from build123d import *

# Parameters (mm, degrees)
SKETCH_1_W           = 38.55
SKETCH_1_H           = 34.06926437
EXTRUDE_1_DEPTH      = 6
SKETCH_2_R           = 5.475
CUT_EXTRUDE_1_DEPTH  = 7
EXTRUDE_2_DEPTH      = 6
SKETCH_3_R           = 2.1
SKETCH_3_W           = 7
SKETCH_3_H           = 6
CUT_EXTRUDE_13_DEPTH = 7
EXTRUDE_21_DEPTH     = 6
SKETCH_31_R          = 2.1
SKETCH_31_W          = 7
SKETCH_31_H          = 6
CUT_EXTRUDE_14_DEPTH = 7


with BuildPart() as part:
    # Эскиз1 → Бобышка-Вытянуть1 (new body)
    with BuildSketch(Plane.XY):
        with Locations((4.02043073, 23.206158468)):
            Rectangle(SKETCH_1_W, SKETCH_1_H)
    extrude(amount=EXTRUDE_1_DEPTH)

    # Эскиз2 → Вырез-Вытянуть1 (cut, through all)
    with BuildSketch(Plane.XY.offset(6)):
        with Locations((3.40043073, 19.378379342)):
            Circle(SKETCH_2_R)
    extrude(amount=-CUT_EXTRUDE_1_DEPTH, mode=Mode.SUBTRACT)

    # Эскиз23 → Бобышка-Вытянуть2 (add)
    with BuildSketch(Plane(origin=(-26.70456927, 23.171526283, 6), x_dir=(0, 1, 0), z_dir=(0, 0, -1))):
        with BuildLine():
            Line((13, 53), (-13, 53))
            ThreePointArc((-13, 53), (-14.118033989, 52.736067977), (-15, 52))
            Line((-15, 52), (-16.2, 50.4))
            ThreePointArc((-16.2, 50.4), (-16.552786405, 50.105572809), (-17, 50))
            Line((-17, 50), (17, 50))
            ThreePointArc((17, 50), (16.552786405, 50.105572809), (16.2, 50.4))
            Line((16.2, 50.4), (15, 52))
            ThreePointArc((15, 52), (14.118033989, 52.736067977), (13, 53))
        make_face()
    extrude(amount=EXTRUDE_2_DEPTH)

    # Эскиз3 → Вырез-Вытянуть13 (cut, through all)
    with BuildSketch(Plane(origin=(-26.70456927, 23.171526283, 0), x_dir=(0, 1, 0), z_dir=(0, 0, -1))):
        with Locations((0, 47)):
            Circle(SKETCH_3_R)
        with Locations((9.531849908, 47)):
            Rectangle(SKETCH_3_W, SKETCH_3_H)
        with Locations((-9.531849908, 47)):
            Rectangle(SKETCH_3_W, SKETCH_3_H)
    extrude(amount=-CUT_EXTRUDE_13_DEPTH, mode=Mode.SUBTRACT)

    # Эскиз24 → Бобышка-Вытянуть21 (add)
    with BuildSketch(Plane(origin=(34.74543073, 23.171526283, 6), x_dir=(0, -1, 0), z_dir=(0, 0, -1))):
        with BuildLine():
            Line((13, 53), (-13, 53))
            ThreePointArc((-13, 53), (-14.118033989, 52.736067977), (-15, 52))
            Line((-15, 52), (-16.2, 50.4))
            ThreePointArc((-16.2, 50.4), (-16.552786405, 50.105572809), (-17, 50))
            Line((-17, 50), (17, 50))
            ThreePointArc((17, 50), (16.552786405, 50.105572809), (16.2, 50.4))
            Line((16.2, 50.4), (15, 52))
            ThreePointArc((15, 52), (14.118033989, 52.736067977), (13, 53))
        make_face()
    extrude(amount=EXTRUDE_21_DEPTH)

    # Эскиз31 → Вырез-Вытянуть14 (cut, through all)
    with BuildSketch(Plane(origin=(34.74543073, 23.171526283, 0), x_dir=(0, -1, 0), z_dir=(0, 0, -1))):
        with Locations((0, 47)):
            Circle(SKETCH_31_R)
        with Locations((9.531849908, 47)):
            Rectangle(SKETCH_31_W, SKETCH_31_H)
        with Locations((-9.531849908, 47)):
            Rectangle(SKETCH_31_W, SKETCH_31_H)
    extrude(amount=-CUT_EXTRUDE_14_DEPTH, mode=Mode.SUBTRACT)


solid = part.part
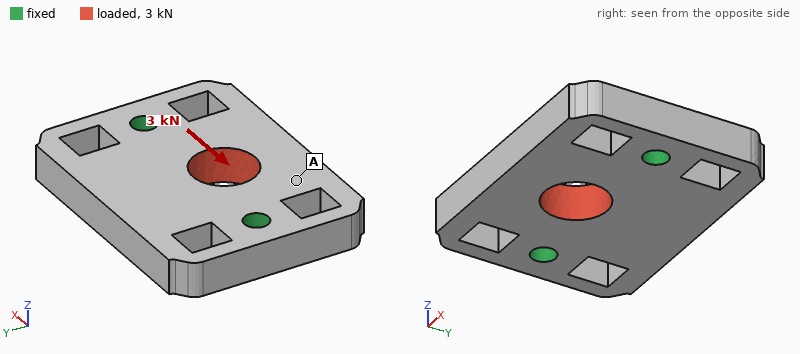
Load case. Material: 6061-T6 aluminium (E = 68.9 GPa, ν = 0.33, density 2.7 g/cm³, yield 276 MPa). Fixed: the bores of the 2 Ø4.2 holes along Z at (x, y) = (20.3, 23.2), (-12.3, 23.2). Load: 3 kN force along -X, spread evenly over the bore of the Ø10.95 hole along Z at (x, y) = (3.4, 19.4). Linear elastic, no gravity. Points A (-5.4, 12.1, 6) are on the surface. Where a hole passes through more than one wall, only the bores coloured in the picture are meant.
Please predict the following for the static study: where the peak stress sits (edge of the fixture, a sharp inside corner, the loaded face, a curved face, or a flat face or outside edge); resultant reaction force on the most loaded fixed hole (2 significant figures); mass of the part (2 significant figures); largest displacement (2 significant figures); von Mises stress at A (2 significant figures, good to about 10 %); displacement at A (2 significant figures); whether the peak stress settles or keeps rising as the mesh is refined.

edge of the fixture
1.5 kN
20 g
7.5 µm
5.5 MPa
5.9 µm
keeps rising
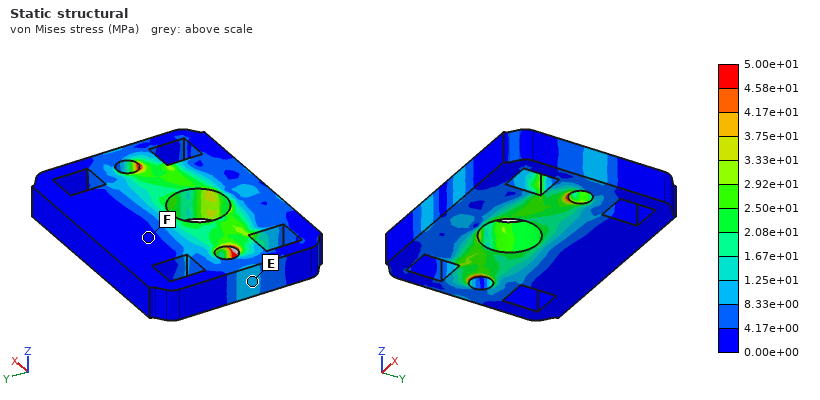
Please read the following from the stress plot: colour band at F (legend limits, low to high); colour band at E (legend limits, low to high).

0.00e+00 to 4.17e+00 MPa
8.33e+00 to 1.25e+01 MPa
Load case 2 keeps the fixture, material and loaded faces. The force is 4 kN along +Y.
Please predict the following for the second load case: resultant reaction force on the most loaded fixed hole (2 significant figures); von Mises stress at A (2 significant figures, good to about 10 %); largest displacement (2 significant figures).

2.1 kN
23 MPa
12 µm
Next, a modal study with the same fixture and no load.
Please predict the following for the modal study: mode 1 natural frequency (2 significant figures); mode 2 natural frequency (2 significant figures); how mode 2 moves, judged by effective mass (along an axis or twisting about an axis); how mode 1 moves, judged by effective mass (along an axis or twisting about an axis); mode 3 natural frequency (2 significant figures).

10 kHz
13 kHz
along Z
twisting about X
19 kHz
